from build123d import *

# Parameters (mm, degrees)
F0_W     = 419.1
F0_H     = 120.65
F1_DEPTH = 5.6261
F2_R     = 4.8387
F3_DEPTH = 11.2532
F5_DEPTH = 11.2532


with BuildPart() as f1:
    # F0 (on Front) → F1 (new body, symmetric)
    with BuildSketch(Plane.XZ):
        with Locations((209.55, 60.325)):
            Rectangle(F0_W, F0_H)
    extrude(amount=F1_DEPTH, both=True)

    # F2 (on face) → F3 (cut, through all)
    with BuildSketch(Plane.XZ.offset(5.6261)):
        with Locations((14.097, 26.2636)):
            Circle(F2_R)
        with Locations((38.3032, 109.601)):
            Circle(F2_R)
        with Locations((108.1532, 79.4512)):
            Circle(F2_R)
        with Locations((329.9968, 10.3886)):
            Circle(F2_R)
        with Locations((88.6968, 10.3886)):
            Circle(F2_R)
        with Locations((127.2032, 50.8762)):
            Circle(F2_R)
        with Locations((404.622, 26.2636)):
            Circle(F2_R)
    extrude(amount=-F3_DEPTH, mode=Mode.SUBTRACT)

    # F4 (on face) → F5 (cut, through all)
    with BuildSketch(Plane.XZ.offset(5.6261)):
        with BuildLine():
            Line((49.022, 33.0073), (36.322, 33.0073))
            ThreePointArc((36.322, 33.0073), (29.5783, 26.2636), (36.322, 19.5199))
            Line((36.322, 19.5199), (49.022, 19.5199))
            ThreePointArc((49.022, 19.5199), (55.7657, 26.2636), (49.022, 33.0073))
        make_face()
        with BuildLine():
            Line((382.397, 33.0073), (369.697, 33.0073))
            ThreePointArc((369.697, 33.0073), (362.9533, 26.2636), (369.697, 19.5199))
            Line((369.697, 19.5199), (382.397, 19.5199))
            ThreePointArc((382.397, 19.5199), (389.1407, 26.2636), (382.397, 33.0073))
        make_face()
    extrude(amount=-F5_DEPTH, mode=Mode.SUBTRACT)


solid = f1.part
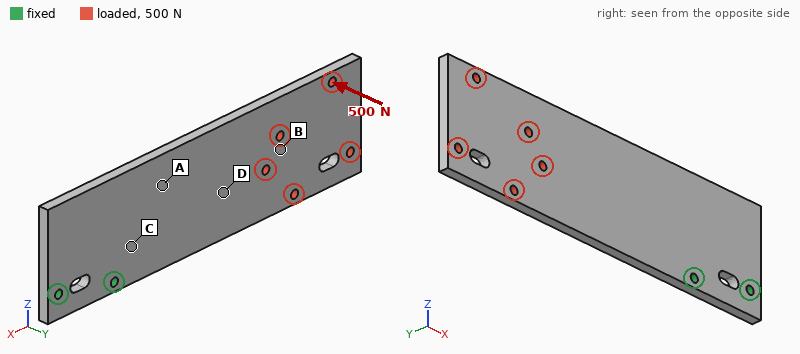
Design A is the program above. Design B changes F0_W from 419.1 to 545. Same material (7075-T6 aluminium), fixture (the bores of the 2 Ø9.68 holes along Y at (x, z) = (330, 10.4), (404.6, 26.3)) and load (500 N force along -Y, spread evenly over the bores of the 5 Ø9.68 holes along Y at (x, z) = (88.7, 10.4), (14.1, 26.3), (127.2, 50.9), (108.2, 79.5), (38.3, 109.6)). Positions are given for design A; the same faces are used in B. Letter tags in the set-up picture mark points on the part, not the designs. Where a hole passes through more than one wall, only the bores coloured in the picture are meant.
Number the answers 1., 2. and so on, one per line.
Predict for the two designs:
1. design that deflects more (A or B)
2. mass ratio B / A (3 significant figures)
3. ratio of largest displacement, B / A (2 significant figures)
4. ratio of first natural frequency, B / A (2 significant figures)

1. B
2. 1.31
3. 1.2
4. 0.71
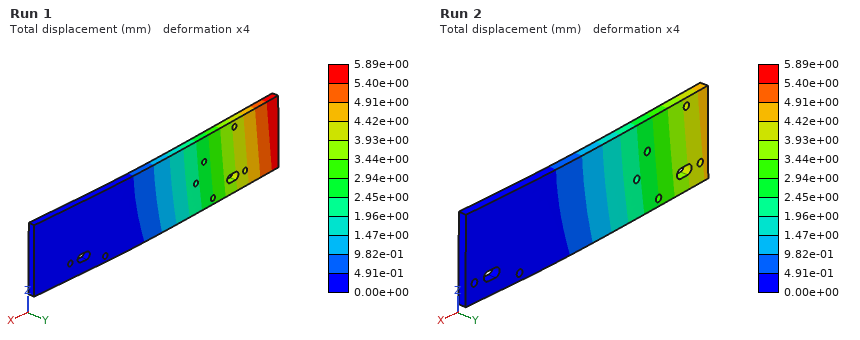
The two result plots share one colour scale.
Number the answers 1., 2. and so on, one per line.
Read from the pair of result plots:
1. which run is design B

1. Run 1
